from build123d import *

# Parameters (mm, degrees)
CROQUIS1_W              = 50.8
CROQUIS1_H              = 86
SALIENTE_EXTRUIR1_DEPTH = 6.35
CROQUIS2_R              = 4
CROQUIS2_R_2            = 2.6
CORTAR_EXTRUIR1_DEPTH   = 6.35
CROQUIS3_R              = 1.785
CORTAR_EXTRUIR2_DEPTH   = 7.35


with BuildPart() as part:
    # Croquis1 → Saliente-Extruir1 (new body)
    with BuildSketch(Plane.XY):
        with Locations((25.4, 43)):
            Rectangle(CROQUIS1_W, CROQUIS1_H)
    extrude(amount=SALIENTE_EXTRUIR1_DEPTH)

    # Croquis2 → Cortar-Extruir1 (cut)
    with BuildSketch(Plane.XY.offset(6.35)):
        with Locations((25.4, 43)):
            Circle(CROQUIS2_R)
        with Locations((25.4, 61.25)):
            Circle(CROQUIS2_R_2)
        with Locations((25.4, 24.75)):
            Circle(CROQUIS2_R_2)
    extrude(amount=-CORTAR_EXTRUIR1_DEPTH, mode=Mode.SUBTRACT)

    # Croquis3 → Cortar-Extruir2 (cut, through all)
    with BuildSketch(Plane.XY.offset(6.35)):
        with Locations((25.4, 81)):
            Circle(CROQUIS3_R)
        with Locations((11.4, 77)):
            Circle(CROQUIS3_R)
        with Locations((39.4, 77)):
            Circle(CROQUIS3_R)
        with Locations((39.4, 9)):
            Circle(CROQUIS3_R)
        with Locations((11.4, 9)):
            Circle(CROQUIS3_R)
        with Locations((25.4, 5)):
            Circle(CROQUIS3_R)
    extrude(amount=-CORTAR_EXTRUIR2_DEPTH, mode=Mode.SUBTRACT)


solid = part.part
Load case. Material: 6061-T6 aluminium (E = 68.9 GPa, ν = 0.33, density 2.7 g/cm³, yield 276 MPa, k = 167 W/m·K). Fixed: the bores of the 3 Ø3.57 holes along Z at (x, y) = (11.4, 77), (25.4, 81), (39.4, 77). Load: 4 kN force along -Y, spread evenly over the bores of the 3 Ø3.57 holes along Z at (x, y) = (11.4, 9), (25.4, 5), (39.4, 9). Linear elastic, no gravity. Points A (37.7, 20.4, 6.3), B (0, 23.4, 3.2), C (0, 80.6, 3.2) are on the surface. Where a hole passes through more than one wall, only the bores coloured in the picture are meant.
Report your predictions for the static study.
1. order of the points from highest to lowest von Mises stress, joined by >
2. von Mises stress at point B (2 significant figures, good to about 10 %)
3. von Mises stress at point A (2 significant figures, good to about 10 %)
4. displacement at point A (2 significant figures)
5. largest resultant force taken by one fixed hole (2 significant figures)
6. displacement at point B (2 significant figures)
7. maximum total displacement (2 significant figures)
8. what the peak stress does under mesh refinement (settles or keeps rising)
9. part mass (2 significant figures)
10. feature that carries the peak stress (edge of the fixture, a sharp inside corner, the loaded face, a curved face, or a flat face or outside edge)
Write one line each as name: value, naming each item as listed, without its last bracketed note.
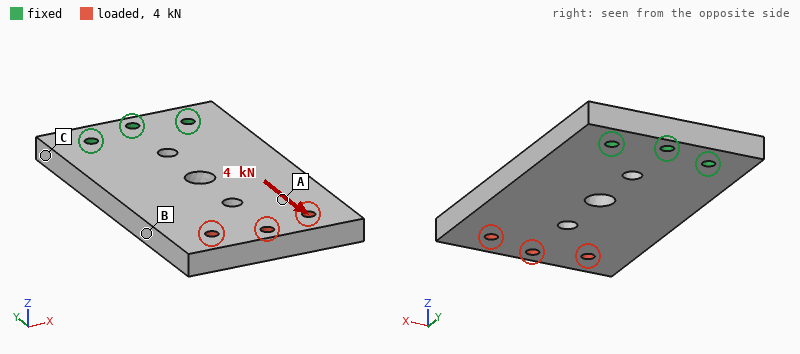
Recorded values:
order of the points from highest to lowest von Mises stress, joined by >: A > B > C
von Mises stress at point B: 8.7 MPa
von Mises stress at point A: 15 MPa
displacement at point A: 12 µm
largest resultant force taken by one fixed hole: 1.6 kN
displacement at point B: 11 µm
maximum total displacement: 18 µm
what the peak stress does under mesh refinement: keeps rising
part mass: 72 g
feature that carries the peak stress: edge of the fixture
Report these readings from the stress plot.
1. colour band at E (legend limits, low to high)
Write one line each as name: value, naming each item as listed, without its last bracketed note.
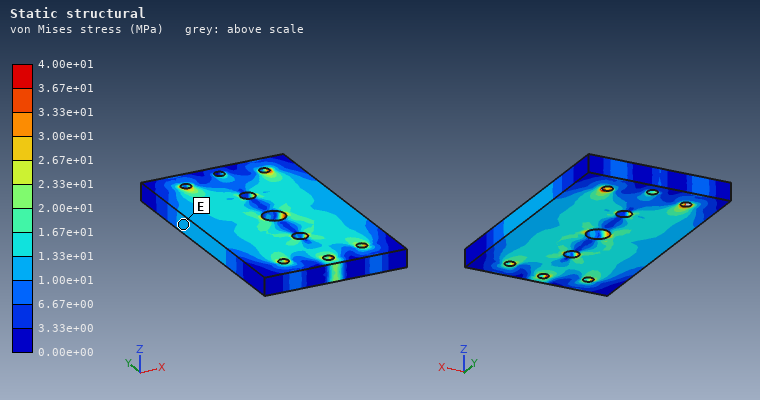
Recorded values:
colour band at E: 1.00e+01 to 1.33e+01 MPa
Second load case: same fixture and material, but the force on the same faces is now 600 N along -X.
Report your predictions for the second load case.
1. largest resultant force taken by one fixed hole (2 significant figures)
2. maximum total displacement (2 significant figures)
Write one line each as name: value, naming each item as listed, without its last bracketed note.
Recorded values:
largest resultant force taken by one fixed hole: 1.4 kN
maximum total displacement: 33 µm
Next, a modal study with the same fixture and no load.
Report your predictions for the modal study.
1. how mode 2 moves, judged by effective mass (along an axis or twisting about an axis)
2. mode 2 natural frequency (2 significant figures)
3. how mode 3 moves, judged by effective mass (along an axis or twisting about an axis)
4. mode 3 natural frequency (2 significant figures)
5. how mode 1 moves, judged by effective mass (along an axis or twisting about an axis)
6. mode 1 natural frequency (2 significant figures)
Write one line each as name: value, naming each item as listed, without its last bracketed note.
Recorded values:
how mode 2 moves, judged by effective mass: twisting about Y
mode 2 natural frequency: 2700 Hz
how mode 3 moves, judged by effective mass: along X
mode 3 natural frequency: 4500 Hz
how mode 1 moves, judged by effective mass: along Z
mode 1 natural frequency: 850 Hz
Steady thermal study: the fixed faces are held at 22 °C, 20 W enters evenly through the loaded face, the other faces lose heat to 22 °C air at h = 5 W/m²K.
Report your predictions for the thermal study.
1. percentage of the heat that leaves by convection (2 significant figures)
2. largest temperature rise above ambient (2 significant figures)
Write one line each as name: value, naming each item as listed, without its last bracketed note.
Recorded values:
percentage of the heat that leaves by convection: 3.6 %
largest temperature rise above ambient: 29 K
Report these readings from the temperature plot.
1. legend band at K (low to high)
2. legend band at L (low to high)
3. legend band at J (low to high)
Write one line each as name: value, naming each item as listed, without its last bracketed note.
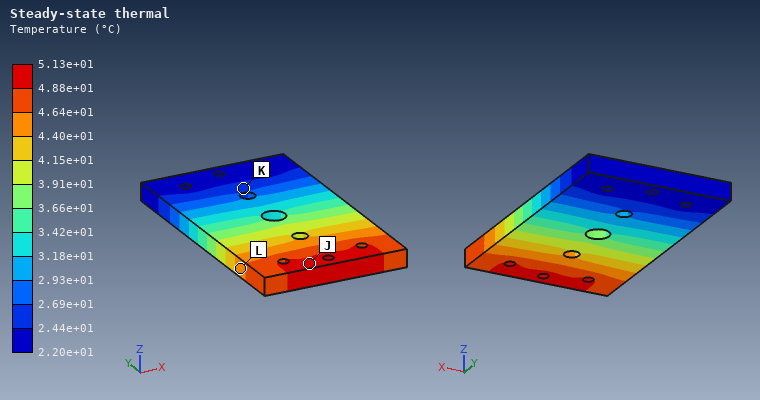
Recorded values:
legend band at K: 2.44e+01 to 2.69e+01 °C
legend band at L: 4.40e+01 to 4.64e+01 °C
legend band at J: 4.88e+01 to 5.13e+01 °C
